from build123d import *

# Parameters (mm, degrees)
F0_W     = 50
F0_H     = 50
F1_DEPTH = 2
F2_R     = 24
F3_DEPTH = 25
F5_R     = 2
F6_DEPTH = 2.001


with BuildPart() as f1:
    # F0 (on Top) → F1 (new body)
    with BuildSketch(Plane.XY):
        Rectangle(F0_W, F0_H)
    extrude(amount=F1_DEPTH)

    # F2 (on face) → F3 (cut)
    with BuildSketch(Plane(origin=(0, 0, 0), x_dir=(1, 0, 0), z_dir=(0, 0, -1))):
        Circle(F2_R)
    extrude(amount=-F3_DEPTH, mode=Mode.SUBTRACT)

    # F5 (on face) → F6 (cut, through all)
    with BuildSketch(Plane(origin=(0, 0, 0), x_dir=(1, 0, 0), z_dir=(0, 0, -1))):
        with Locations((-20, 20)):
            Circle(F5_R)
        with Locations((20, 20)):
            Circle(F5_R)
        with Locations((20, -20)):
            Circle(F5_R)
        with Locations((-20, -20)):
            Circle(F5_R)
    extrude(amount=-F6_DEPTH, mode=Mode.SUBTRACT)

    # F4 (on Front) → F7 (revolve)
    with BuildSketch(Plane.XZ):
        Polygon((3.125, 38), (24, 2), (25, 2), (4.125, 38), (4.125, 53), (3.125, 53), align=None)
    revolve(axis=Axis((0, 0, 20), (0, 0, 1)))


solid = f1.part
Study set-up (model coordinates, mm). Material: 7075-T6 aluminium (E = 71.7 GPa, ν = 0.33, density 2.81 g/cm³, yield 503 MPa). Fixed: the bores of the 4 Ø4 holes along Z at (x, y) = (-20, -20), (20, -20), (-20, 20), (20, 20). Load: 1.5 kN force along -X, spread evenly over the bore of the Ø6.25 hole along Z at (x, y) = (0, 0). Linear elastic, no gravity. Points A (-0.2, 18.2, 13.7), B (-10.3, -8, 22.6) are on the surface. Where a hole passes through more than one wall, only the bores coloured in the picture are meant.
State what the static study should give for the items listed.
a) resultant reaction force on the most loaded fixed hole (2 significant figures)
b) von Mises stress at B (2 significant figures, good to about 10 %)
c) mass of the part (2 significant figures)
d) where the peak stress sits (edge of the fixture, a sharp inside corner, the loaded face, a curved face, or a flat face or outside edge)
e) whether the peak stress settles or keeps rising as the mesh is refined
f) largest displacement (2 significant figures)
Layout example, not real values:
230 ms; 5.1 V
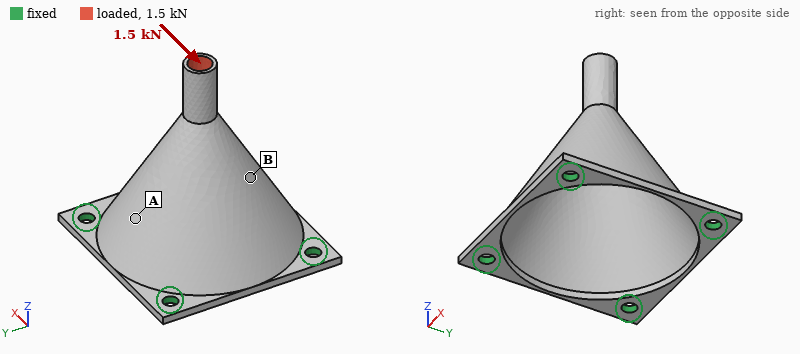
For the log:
1.1 kN; 82 MPa; 13 g; a sharp inside corner; keeps rising; 0.38 mm
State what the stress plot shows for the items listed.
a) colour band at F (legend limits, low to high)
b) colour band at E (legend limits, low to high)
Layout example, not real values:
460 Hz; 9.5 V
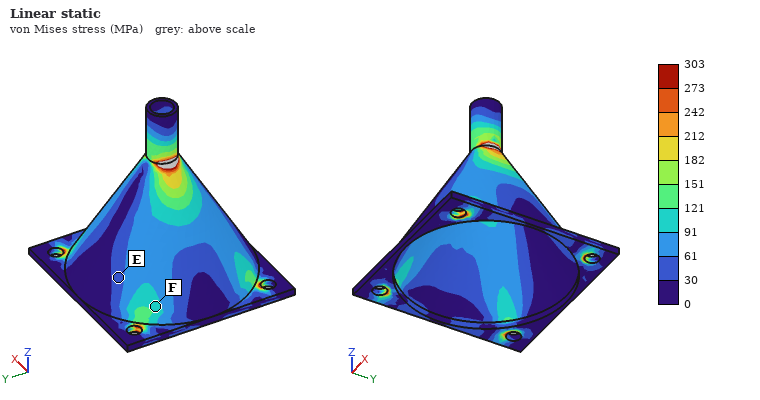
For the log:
91 to 121 MPa; 30 to 61 MPa
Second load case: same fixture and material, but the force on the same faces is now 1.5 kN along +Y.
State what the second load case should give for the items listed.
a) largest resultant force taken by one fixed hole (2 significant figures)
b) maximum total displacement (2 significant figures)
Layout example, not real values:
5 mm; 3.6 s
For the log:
1.1 kN; 0.38 mm
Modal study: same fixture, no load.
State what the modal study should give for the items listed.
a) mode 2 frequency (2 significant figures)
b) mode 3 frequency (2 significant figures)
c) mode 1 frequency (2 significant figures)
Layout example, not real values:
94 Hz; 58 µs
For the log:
9500 Hz; 11 kHz; 9500 Hz
